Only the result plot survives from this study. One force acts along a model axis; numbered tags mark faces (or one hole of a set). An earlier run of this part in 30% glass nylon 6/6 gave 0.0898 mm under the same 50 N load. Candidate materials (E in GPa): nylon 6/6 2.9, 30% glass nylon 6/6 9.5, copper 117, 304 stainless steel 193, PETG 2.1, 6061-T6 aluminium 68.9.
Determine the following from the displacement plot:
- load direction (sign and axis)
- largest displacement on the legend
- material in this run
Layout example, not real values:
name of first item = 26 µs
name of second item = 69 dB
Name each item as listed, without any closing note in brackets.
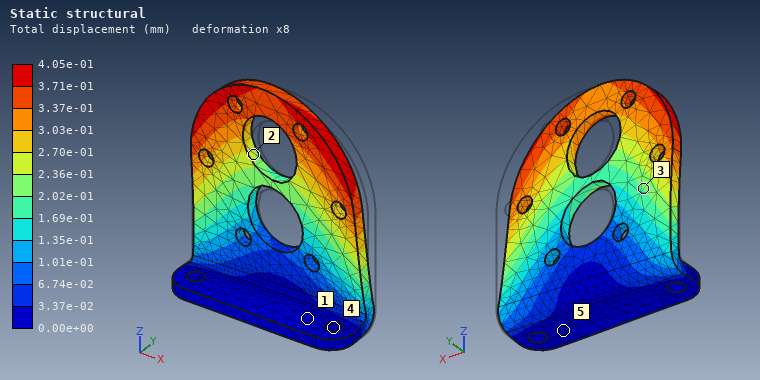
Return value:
load direction = -X
largest displacement on the legend = 4.05e-01 mm
material in this run = PETG
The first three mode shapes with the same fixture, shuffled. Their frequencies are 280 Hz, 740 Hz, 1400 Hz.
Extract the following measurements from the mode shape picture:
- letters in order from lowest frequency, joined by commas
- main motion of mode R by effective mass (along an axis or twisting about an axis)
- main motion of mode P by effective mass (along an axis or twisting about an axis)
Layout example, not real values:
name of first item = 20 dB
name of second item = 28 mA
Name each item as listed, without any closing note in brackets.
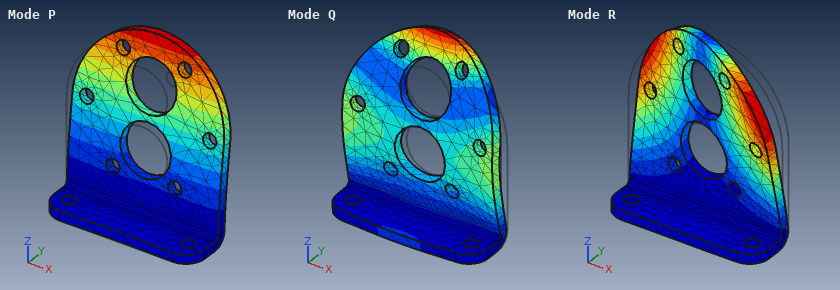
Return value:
letters in order from lowest frequency, joined by commas = P, R, Q
main motion of mode R by effective mass = twisting about Z
main motion of mode P by effective mass = along Y
